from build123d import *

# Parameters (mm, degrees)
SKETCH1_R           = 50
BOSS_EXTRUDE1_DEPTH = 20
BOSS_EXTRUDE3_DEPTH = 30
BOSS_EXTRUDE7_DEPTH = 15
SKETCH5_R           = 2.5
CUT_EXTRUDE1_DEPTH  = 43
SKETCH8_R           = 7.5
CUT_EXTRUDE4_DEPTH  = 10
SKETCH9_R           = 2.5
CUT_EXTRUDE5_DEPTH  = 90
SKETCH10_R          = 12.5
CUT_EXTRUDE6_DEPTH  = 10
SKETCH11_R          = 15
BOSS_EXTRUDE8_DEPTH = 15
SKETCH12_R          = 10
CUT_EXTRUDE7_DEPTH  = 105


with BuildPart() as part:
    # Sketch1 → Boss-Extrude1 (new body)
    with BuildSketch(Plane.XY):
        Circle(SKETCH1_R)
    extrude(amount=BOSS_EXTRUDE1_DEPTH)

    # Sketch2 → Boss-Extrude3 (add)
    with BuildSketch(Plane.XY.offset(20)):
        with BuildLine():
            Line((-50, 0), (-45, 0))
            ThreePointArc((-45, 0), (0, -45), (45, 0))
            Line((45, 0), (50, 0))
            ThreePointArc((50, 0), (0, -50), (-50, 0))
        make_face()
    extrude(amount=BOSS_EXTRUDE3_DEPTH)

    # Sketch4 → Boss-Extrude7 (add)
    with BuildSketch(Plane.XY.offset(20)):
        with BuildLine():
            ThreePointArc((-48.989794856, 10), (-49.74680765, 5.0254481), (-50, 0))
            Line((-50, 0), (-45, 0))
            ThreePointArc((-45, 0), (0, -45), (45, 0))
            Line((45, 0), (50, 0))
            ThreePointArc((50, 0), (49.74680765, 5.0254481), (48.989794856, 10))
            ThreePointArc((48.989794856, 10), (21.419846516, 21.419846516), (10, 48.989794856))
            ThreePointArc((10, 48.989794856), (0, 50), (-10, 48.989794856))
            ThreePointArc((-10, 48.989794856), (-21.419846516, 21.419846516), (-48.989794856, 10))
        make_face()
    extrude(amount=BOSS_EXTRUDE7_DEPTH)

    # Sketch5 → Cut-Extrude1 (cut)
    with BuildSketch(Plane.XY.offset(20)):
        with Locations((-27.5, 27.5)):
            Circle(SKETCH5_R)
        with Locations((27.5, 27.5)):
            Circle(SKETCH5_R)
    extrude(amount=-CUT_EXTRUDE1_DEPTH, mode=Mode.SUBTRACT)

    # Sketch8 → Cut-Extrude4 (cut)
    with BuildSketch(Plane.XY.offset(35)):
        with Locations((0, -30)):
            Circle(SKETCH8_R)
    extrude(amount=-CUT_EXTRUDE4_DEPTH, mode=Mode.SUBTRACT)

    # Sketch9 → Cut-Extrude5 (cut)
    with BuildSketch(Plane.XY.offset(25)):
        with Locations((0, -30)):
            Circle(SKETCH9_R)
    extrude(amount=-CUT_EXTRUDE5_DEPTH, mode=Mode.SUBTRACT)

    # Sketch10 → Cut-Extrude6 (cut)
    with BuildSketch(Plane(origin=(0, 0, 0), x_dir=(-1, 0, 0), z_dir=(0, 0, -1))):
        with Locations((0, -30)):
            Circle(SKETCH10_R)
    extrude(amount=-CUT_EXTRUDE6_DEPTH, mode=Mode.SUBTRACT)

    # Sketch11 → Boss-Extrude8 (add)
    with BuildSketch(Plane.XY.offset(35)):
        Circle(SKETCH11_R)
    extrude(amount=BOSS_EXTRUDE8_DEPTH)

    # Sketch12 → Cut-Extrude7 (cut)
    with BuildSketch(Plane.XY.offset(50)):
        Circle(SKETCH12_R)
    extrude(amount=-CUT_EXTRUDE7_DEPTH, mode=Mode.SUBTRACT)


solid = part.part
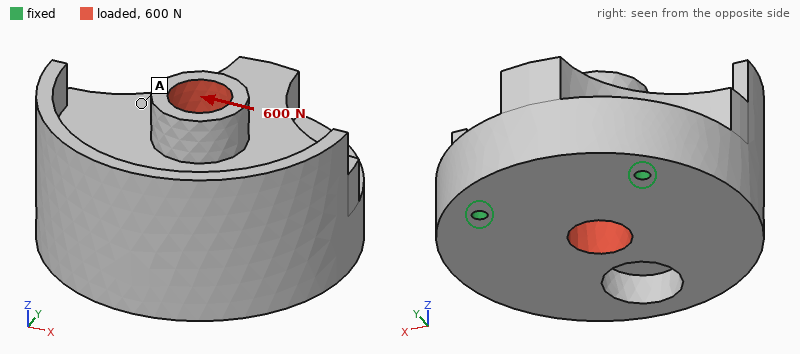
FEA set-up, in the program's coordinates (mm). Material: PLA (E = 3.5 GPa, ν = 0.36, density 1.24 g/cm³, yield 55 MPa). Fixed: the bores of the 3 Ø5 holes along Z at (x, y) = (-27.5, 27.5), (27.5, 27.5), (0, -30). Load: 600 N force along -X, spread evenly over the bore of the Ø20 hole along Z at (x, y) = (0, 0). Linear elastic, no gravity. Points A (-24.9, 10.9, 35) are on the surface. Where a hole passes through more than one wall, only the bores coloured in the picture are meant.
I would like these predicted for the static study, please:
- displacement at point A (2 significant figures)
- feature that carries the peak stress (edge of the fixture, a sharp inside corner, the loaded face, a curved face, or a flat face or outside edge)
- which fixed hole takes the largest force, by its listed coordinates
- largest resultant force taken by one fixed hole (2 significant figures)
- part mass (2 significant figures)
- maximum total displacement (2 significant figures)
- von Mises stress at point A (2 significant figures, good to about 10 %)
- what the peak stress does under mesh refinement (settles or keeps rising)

6.9 µm
edge of the fixture
(0, -30)
250 N
310 g
18 µm
0.27 MPa
keeps rising
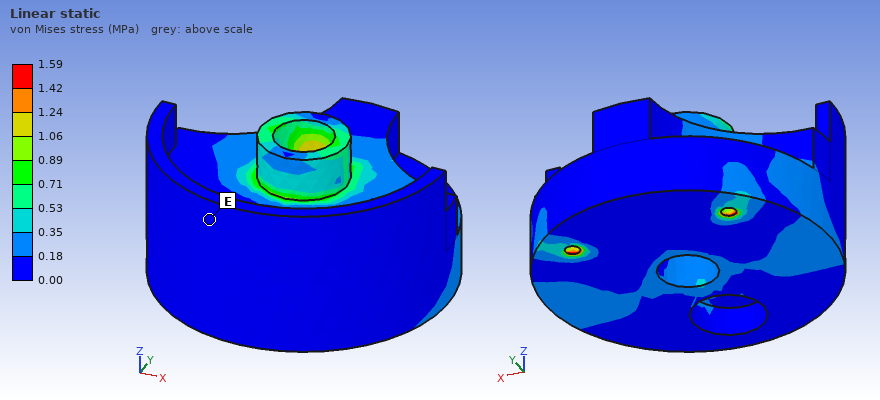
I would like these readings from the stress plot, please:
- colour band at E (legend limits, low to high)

0.00 to 0.18 MPa
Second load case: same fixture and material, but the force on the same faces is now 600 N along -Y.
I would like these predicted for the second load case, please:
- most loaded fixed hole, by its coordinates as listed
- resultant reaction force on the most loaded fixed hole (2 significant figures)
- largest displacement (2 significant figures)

(0, -30)
270 N
15 µm
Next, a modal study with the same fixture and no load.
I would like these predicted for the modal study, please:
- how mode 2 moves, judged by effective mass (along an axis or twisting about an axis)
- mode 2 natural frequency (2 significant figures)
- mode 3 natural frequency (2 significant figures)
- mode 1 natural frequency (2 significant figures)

along Z
2700 Hz
3800 Hz
2000 Hz
